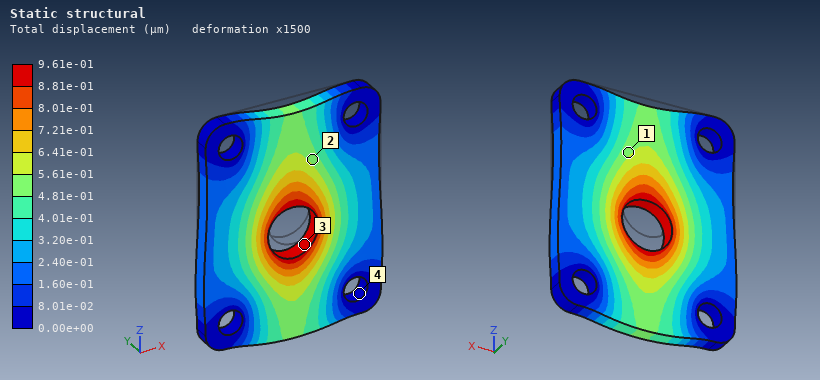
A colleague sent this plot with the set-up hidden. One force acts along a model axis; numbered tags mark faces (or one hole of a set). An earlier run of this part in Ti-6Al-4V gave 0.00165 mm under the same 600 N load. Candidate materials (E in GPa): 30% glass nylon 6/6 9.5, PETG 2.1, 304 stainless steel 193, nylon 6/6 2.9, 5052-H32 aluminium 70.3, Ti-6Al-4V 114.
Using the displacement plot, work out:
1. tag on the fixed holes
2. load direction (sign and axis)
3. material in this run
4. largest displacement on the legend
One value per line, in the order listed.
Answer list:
4
-Z
304 stainless steel
9.61e-01 µm
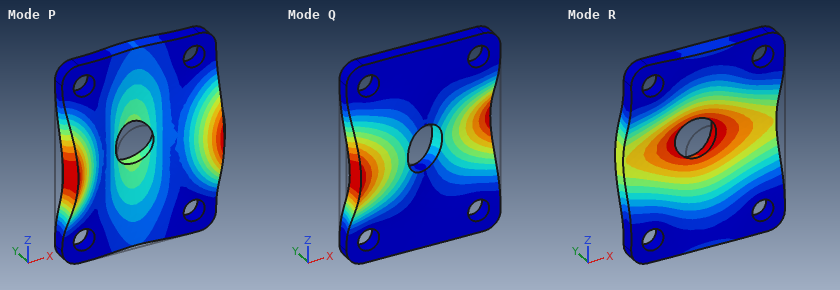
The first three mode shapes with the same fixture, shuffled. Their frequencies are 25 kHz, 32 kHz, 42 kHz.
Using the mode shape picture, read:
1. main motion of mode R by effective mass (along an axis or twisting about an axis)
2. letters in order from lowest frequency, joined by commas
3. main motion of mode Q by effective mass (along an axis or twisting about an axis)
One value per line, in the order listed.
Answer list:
along Y
R, Q, P
twisting about Z
